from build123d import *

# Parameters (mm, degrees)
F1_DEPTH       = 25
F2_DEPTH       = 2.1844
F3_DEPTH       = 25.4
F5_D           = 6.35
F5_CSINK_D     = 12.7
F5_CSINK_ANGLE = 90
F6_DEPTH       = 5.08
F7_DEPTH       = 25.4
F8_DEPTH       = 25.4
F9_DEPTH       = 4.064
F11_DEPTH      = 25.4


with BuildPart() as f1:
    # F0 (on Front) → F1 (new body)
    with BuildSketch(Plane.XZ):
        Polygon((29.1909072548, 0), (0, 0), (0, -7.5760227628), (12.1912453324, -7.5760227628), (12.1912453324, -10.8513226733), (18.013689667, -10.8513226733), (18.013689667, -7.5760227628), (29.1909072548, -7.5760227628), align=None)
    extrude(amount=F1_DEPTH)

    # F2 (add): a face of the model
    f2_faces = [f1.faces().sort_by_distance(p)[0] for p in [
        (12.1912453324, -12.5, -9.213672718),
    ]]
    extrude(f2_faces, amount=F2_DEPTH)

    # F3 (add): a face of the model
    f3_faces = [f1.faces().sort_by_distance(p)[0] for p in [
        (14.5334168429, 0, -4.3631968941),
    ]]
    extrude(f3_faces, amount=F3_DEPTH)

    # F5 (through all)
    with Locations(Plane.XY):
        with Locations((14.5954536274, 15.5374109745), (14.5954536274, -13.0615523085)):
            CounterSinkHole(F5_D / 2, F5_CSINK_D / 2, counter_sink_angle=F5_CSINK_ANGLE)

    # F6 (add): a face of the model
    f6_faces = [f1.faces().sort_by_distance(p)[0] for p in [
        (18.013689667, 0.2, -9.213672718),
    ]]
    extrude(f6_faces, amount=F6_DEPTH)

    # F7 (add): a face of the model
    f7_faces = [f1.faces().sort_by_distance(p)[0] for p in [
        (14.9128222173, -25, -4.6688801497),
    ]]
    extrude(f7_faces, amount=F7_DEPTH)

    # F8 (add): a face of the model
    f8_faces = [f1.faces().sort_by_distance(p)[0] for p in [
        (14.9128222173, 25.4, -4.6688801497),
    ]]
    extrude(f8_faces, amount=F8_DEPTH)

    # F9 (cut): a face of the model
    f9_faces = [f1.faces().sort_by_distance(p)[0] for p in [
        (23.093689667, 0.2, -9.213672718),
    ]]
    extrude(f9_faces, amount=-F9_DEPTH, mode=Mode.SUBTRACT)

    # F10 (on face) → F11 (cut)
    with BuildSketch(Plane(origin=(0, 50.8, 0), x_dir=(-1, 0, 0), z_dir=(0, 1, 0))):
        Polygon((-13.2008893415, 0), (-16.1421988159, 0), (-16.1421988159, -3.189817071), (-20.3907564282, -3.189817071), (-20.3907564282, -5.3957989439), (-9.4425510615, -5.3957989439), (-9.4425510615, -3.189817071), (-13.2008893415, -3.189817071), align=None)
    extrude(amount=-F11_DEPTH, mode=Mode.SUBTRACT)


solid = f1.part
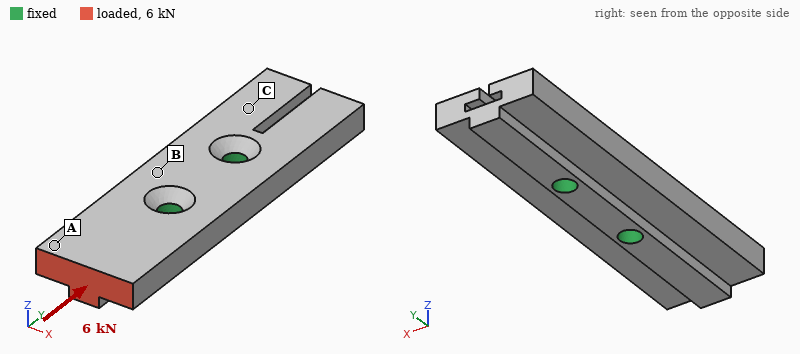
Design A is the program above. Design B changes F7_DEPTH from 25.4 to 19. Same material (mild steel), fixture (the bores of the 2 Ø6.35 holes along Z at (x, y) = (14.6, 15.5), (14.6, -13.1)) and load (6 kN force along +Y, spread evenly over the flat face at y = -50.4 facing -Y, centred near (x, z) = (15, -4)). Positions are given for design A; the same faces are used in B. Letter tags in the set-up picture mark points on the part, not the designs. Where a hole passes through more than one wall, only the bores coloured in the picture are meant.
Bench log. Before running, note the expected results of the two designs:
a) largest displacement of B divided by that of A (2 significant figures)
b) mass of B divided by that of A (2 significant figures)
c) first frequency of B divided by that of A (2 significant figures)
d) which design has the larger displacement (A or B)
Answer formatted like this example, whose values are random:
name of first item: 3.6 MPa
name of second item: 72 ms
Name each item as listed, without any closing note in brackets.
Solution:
largest displacement of B divided by that of A: 0.84
mass of B divided by that of A: 0.93
first frequency of B divided by that of A: 1.1
which design has the larger displacement: A
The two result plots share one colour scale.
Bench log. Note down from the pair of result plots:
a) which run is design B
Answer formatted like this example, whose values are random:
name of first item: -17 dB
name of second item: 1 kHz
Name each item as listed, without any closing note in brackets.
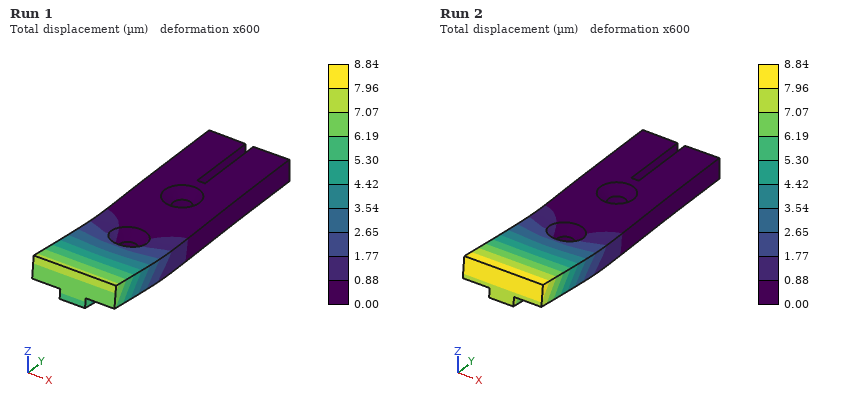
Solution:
which run is design B: Run 1
